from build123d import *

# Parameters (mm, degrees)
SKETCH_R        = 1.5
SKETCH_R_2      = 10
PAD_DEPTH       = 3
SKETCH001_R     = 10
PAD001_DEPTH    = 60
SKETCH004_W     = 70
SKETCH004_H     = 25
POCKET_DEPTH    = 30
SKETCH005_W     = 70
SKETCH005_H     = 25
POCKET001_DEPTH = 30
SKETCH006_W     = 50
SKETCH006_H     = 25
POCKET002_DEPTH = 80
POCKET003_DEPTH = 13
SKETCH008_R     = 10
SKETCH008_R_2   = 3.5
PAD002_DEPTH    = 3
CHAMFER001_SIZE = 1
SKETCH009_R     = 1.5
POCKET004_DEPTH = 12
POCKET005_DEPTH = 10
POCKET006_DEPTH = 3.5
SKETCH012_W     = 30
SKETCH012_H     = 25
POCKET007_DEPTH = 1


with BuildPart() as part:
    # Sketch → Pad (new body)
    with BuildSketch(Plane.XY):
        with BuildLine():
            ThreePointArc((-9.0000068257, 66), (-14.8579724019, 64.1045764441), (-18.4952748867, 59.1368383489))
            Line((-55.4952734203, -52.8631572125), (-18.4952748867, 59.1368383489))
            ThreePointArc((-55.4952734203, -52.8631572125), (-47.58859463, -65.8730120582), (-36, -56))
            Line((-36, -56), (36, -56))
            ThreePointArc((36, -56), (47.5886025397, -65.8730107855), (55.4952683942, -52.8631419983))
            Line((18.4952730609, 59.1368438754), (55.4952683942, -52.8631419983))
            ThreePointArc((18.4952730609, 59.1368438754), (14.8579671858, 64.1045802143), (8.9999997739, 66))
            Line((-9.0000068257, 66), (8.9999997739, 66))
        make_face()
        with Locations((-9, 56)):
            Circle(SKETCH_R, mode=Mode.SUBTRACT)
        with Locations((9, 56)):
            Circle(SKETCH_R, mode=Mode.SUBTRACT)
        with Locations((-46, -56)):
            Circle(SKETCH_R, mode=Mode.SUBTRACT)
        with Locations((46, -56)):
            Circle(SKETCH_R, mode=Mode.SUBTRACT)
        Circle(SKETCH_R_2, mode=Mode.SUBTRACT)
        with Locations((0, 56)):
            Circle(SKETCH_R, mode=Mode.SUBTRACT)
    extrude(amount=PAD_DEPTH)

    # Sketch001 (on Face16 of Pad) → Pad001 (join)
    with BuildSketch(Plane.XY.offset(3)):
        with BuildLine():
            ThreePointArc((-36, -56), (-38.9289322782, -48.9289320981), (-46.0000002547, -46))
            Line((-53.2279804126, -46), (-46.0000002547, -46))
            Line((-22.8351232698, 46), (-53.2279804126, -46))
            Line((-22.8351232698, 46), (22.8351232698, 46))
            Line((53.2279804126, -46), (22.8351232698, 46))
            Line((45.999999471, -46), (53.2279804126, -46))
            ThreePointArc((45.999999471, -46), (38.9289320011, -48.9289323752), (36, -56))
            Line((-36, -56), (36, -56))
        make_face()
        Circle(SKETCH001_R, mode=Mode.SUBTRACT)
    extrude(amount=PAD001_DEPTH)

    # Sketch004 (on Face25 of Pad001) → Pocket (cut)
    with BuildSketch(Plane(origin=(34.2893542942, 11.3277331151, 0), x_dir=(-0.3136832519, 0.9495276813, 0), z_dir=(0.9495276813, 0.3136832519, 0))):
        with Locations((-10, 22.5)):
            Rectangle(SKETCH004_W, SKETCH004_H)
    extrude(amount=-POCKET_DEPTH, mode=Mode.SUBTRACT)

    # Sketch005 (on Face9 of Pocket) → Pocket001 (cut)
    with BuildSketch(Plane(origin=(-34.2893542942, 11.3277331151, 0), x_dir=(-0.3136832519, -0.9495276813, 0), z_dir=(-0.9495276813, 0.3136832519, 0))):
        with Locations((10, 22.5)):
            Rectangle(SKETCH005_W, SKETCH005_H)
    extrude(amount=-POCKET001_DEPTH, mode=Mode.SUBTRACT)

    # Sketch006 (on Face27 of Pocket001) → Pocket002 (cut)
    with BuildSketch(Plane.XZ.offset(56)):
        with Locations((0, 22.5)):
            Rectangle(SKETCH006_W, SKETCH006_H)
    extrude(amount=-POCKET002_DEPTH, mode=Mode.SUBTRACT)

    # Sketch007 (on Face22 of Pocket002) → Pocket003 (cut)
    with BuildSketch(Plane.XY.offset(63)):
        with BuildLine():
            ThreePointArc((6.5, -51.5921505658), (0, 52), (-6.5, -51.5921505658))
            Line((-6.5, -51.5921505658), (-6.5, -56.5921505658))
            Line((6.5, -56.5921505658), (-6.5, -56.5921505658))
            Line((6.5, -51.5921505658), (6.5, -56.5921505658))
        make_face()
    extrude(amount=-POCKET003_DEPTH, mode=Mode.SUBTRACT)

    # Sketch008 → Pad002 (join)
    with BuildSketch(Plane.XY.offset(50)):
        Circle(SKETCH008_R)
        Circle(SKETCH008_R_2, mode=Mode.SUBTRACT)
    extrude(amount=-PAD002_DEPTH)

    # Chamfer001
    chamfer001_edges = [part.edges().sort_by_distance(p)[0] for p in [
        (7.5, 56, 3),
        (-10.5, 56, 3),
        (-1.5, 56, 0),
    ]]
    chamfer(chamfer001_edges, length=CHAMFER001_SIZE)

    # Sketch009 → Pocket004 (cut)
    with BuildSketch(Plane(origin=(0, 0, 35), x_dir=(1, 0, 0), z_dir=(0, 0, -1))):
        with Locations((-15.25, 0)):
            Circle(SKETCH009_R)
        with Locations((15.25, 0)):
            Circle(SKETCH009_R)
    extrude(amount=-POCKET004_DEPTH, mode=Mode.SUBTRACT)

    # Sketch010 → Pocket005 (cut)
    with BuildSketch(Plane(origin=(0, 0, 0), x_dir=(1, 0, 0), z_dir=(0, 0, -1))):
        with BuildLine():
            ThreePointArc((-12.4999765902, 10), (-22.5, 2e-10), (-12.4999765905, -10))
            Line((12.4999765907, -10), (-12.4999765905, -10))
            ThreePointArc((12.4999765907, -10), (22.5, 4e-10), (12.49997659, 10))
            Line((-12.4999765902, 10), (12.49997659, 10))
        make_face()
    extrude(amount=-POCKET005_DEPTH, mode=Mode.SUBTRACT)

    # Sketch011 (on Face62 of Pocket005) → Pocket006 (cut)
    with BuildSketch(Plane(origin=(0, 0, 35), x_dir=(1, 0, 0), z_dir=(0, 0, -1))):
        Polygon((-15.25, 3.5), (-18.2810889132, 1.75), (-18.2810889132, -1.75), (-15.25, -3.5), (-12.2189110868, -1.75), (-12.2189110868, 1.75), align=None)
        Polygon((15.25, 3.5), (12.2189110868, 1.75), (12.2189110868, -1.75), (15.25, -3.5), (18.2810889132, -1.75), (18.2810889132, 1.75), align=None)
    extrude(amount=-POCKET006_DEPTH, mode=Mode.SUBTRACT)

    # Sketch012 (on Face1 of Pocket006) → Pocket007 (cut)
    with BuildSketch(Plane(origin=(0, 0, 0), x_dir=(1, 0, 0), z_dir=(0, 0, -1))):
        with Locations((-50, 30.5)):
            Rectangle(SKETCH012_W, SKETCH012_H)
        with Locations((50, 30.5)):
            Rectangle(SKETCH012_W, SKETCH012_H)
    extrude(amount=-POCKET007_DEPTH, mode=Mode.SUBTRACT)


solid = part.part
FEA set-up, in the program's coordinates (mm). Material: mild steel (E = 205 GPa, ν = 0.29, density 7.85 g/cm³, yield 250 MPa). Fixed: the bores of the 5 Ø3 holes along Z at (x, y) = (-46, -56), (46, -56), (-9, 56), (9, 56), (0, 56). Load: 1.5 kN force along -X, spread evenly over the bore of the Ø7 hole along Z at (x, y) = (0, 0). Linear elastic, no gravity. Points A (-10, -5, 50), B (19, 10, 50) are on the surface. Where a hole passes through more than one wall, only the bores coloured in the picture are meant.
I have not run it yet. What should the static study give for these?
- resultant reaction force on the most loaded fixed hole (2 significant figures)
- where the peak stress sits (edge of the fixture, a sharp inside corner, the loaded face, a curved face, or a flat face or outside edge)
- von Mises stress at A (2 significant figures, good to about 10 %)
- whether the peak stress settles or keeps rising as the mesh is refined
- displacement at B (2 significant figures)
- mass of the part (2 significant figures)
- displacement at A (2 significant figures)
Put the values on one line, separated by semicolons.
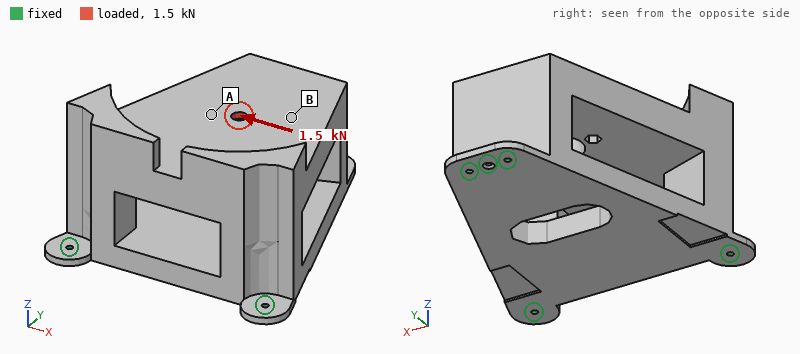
1.0 kN; edge of the fixture; 14 MPa; keeps rising; 17 µm; 1.9 kg; 16 µm
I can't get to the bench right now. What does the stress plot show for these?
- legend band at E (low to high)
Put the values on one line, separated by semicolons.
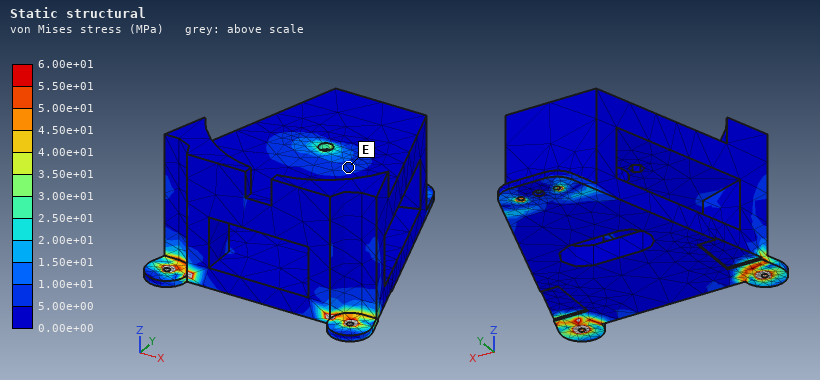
5.00e+00 to 1.00e+01 MPa
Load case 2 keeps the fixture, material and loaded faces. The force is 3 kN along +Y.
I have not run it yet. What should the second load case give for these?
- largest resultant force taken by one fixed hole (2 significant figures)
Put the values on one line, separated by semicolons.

1000 N
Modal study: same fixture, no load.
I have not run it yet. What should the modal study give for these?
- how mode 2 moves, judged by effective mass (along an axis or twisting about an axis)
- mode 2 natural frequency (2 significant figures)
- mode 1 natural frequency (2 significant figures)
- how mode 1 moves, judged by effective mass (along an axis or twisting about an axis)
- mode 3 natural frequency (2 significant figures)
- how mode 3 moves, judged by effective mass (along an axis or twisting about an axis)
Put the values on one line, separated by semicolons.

along Z; 1800 Hz; 1400 Hz; along X; 1900 Hz; along Y
